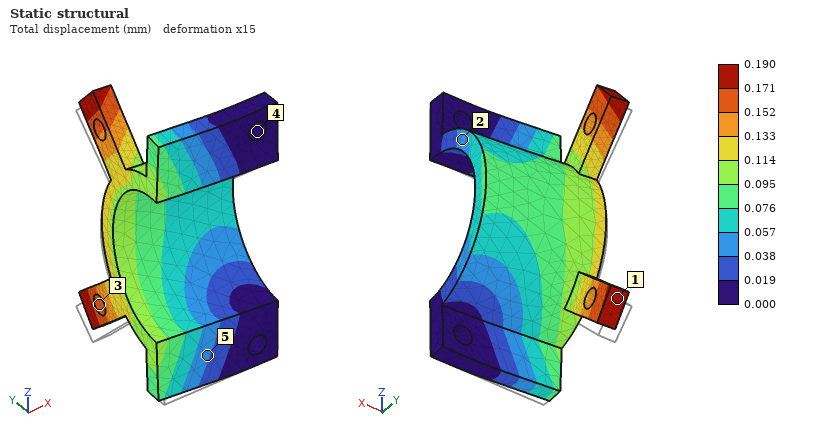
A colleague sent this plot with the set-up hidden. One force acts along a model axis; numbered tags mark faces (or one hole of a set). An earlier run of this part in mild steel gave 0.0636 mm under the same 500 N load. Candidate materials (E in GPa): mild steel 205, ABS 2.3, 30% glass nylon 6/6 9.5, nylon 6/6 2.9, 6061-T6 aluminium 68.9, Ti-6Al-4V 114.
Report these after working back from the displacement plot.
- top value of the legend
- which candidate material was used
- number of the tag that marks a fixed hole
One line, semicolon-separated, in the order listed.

0.190 mm; 6061-T6 aluminium; 4
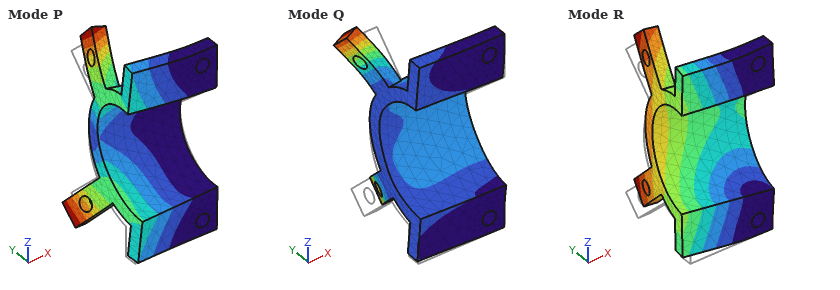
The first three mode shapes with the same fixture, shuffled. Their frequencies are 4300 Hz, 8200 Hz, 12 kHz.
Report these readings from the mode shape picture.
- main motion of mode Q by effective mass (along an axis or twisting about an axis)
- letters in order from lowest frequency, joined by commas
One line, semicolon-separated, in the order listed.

along Z; R, P, Q
